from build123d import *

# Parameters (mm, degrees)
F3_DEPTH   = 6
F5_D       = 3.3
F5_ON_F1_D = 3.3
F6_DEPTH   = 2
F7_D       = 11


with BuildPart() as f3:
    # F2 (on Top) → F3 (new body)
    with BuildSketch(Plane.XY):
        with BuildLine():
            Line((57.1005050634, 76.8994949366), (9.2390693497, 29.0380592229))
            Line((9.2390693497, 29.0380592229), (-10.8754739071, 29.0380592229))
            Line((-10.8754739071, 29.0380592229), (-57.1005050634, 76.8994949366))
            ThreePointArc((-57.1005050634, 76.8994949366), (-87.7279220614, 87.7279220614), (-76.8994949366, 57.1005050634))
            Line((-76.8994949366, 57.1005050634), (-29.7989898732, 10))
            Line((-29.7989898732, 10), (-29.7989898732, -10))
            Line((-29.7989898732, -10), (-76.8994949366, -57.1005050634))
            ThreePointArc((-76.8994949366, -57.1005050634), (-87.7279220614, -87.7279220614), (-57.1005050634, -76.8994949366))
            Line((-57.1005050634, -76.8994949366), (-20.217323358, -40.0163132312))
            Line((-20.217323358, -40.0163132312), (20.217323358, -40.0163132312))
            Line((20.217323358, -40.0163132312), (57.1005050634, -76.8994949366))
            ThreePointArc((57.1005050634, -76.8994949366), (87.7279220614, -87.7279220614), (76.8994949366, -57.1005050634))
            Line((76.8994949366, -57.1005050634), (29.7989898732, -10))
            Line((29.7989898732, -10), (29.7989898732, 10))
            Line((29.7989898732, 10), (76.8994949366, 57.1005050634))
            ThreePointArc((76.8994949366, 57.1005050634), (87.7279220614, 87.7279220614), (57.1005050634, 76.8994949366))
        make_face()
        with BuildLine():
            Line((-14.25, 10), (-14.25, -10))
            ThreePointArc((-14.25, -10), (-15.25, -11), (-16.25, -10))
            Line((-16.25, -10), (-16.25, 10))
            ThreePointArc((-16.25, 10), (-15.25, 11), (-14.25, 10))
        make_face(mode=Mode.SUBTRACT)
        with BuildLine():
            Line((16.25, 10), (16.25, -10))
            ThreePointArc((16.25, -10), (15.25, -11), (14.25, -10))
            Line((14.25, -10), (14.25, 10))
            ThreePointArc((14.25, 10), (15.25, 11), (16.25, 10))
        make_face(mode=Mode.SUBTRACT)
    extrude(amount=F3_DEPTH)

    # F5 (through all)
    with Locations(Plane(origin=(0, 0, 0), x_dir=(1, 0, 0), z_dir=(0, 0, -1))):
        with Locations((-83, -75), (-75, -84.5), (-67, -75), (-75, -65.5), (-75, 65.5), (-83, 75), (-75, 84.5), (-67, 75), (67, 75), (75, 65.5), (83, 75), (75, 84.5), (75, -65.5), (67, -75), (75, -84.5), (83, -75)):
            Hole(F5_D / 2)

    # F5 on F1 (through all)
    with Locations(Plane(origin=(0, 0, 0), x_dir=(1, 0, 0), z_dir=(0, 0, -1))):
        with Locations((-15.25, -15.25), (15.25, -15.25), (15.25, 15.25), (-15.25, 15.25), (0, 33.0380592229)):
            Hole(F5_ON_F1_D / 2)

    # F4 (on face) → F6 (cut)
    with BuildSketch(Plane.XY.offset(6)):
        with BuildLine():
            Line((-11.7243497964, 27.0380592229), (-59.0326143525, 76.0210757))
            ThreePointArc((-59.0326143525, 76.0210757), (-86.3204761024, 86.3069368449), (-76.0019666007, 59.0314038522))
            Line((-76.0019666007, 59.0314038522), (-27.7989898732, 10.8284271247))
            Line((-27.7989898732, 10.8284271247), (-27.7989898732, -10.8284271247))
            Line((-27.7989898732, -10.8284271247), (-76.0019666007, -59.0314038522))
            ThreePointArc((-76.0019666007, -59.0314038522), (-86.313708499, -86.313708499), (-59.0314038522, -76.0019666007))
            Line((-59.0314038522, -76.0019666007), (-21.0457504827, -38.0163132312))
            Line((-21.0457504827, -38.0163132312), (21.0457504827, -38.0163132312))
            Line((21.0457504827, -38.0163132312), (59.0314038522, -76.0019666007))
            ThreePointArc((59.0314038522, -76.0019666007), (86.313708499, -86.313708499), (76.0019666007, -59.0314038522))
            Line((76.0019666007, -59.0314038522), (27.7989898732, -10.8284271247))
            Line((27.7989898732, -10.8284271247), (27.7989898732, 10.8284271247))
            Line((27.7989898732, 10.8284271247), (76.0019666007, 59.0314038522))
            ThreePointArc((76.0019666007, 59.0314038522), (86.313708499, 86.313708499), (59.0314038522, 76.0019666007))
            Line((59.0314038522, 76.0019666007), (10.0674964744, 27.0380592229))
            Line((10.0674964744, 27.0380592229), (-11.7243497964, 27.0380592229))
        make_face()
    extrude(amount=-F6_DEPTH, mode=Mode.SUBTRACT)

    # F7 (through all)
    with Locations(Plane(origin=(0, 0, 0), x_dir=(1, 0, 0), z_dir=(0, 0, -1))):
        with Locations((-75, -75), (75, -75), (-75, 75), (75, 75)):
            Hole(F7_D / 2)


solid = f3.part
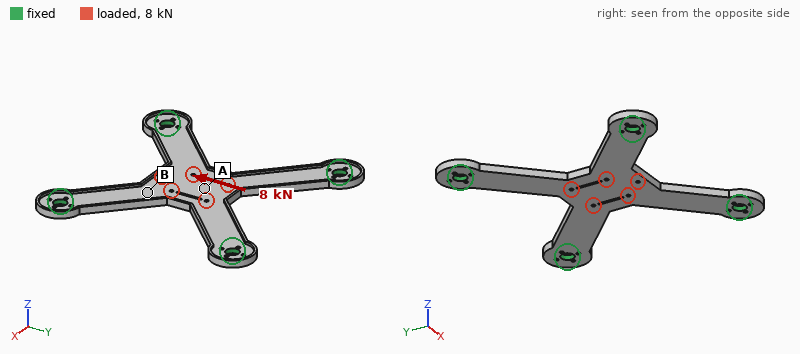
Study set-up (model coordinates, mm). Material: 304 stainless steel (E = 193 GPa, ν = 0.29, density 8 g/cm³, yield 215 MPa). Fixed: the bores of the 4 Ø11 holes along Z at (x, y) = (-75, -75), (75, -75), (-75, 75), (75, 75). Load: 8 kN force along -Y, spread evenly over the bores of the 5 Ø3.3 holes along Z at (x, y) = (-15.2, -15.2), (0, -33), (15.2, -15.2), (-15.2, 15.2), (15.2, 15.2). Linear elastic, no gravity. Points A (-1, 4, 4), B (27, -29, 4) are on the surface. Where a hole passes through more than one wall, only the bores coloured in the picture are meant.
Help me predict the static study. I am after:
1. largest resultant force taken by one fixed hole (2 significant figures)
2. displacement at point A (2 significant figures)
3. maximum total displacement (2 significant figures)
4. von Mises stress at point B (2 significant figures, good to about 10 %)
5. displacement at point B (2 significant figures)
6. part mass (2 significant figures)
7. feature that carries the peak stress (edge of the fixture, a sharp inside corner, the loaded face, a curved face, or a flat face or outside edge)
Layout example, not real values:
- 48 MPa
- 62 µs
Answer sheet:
- 2.7 kN
- 16 µm
- 20 µm
- 21 MPa
- 13 µm
- 460 g
- a curved face
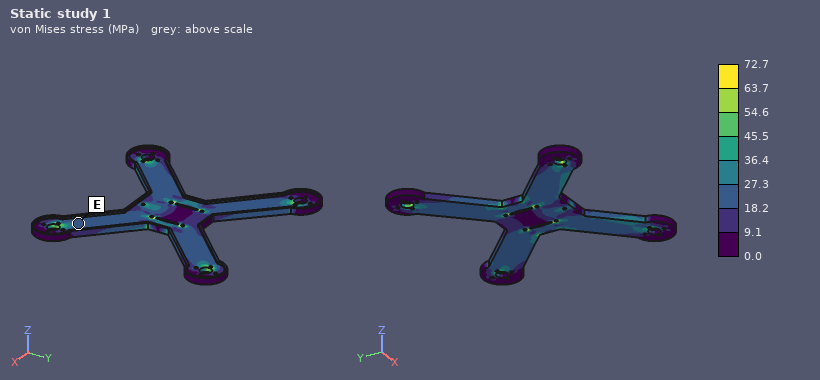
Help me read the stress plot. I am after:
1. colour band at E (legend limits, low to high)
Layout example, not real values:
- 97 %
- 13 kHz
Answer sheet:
- 18.2 to 27.3 MPa
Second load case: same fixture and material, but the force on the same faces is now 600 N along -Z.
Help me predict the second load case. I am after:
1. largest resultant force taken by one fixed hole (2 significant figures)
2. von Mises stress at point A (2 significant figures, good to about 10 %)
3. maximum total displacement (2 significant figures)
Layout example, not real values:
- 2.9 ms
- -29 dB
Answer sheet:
- 170 N
- 29 MPa
- 0.25 mm
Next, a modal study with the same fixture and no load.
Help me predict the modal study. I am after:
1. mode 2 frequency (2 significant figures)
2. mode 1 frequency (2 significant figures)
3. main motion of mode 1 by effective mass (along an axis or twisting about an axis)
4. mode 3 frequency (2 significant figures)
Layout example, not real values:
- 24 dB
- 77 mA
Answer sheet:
- 1500 Hz
- 620 Hz
- along Z
- 1500 Hz
